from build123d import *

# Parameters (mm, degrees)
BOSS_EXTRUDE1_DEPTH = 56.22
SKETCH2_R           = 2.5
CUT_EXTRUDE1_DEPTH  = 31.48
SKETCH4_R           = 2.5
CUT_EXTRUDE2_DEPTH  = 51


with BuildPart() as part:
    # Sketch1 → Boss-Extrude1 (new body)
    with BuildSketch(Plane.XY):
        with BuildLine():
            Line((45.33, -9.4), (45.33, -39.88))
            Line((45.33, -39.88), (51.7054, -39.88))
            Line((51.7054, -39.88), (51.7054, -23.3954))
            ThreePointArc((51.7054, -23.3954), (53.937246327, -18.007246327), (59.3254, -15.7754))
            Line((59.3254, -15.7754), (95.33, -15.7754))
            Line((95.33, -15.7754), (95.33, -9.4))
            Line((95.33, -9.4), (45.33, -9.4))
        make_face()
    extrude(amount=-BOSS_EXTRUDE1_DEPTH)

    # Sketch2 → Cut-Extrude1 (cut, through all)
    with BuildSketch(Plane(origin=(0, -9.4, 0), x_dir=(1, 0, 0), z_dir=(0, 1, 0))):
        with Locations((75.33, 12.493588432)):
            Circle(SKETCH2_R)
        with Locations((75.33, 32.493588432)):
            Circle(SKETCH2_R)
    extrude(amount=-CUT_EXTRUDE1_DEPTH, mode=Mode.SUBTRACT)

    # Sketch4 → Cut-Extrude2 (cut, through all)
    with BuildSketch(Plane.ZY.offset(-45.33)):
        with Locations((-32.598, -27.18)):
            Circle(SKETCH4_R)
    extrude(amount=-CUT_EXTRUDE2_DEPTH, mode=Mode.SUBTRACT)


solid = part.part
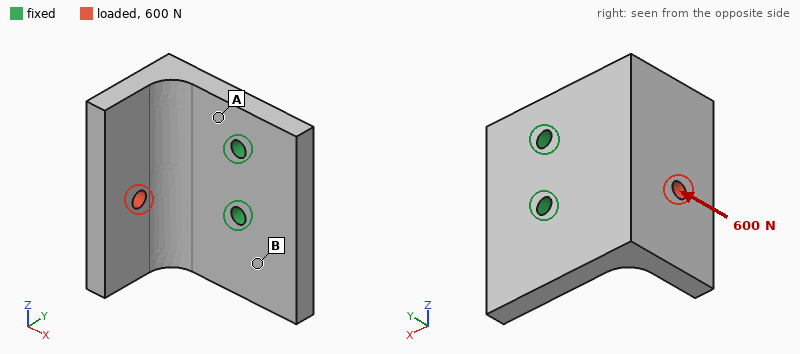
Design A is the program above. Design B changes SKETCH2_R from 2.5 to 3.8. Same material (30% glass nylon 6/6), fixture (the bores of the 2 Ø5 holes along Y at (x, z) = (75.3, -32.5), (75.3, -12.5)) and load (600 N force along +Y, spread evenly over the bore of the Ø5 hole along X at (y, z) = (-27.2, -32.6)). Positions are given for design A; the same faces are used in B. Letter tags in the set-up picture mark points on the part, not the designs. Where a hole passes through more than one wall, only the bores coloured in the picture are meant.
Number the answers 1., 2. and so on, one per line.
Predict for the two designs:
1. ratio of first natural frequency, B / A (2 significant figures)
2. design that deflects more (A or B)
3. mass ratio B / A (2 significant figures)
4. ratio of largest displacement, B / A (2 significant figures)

1. 1.1
2. A
3. 0.99
4. 0.83
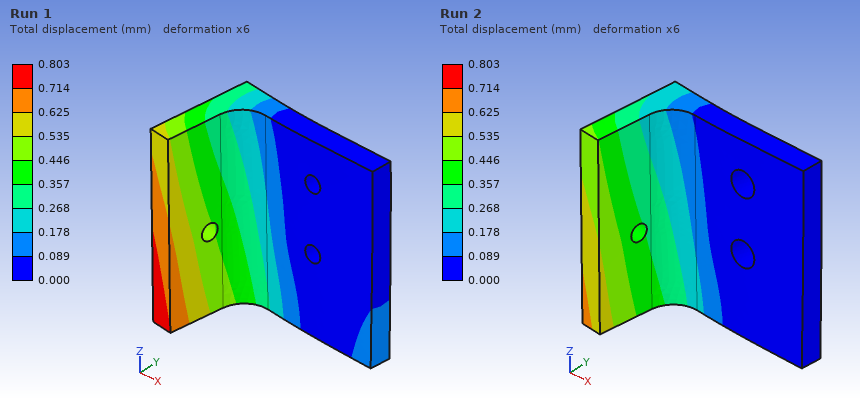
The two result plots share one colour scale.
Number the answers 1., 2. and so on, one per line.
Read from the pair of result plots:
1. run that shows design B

1. Run 2
